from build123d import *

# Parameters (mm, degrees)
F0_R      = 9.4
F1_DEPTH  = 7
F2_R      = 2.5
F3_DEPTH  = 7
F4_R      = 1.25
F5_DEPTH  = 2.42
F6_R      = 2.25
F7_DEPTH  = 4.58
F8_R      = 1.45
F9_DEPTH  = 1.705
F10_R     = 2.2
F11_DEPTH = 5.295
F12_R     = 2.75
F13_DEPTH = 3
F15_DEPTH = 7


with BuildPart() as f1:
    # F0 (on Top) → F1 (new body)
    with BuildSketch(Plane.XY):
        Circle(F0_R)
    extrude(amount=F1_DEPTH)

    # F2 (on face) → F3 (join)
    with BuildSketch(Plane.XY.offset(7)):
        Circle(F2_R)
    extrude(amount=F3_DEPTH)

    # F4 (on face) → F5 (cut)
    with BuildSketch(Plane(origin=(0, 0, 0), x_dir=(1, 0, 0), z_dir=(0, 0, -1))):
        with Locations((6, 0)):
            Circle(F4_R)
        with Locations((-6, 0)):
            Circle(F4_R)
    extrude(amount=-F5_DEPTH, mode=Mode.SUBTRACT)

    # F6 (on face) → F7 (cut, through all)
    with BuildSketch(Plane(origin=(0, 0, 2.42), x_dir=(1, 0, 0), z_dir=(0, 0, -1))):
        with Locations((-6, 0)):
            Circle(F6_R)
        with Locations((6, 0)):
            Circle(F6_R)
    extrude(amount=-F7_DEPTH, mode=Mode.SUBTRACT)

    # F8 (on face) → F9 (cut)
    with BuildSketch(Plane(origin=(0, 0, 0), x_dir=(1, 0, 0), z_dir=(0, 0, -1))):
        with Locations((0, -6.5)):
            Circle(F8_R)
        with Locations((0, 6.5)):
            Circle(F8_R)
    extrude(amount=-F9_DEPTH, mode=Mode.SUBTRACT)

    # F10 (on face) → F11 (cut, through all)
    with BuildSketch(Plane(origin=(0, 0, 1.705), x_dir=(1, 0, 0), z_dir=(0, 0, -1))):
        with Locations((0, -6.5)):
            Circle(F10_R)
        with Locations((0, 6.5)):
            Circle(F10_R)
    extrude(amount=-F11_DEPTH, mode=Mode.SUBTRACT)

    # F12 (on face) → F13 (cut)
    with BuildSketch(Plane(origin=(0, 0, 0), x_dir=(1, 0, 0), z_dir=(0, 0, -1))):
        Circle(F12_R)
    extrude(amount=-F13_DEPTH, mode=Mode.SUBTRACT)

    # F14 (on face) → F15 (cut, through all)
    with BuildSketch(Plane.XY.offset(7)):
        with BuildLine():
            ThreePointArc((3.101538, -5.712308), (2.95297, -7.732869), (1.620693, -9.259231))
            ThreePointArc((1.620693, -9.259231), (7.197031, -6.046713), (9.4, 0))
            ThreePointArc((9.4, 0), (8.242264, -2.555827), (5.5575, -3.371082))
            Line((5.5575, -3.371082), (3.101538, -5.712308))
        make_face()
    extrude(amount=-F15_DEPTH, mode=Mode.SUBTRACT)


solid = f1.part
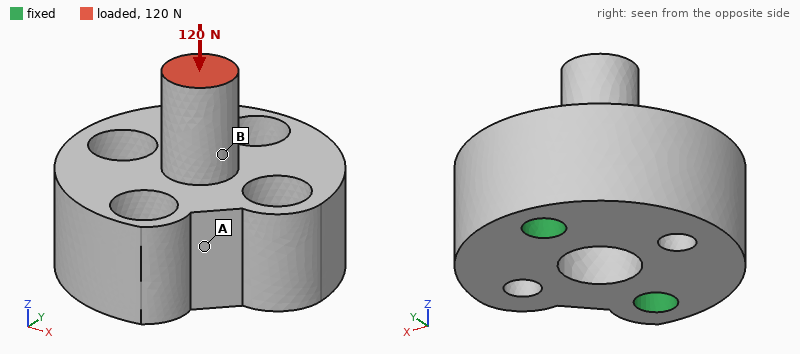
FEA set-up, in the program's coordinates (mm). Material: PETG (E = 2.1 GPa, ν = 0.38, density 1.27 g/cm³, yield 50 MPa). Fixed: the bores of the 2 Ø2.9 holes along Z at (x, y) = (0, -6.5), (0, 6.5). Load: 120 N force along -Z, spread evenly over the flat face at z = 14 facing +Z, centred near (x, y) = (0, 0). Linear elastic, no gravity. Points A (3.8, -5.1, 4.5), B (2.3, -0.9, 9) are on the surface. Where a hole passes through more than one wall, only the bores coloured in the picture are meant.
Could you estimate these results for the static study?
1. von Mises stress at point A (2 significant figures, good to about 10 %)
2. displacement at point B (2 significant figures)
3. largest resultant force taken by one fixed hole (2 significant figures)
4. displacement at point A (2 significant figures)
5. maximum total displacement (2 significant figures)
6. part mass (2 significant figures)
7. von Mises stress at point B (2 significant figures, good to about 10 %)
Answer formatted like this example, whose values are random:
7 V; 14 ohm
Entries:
2.0 MPa; 28 µm; 66 N; 13 µm; 43 µm; 1.9 g; 5.9 MPa
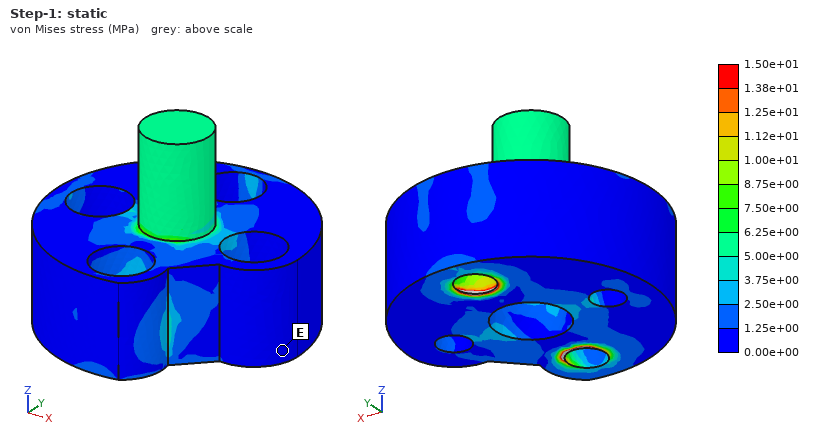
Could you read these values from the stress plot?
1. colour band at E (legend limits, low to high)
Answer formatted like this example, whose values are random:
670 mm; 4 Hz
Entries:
0.00e+00 to 1.25e+00 MPa
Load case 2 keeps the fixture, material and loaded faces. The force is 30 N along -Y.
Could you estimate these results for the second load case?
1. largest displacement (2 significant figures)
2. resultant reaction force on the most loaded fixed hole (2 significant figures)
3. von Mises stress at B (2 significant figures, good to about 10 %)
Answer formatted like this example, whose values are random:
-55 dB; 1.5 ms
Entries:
0.12 mm; 35 N; 5.0 MPa
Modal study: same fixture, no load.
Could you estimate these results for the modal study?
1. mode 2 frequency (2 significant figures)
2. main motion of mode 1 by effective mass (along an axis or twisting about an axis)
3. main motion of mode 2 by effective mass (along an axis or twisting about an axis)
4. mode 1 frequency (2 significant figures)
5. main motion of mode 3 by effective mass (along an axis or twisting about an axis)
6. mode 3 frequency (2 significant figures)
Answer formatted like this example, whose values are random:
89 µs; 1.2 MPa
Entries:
9600 Hz; along X; along Y; 3500 Hz; along Z; 10 kHz
